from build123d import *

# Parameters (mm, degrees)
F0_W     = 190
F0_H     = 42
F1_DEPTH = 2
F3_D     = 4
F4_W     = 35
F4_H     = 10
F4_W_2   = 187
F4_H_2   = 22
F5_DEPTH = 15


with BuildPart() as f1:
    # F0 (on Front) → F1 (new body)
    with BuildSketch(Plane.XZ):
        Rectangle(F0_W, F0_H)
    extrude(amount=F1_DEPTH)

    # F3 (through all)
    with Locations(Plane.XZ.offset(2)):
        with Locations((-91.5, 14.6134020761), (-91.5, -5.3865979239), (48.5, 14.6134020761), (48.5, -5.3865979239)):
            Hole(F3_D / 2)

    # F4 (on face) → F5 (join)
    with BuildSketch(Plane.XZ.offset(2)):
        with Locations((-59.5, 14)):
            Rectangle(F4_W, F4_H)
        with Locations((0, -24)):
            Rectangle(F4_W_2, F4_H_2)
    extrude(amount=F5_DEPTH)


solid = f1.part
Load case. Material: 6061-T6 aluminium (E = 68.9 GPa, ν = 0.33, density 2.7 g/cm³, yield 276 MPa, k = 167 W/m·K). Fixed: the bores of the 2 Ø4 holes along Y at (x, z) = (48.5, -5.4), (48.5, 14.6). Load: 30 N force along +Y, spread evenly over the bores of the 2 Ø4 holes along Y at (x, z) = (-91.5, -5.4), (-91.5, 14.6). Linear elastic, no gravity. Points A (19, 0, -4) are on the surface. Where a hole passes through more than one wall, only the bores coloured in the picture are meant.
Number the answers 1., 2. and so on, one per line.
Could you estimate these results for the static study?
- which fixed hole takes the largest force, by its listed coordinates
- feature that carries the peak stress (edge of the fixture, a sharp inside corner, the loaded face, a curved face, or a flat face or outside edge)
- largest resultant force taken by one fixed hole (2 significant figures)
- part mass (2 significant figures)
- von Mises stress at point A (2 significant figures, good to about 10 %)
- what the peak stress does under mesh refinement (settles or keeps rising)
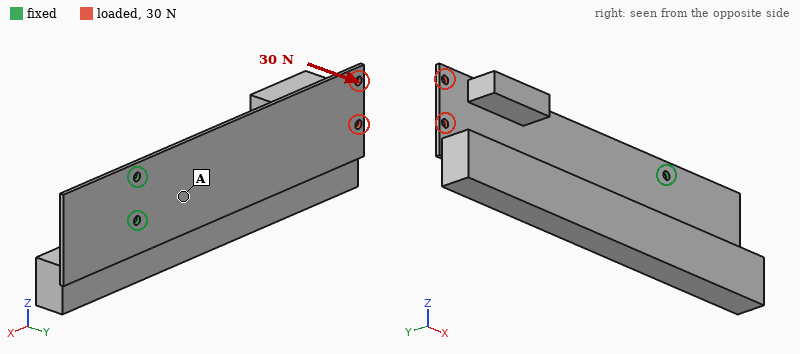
1. (48.5, -5.4)
2. edge of the fixture
3. 19 N
4. 220 g
5. 12 MPa
6. keeps rising
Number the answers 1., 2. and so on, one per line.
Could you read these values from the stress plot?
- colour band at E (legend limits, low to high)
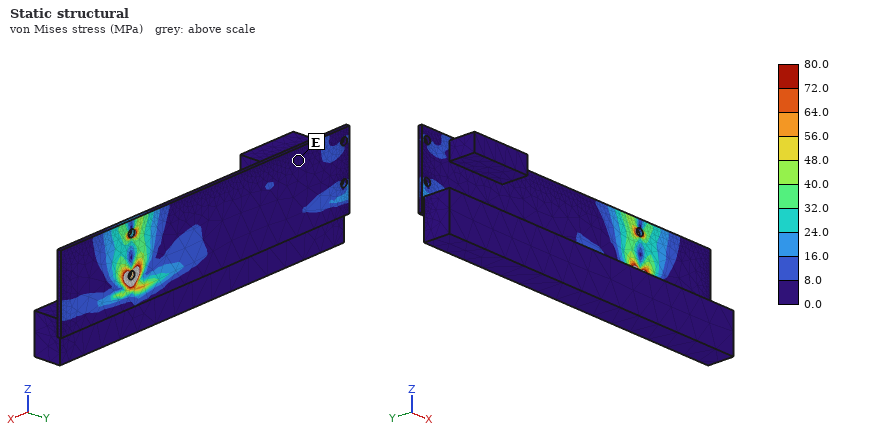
1. 0.0 to 8.0 MPa
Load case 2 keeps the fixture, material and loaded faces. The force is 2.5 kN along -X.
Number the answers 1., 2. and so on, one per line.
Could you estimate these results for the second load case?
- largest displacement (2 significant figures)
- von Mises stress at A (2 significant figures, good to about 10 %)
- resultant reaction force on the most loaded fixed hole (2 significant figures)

1. 0.15 mm
2. 23 MPa
3. 1.3 kN
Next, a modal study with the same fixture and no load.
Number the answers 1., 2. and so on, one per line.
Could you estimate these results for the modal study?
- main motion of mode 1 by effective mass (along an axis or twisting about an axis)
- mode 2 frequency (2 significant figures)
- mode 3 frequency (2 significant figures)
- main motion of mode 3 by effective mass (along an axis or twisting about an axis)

1. along Y
2. 330 Hz
3. 770 Hz
4. along Z
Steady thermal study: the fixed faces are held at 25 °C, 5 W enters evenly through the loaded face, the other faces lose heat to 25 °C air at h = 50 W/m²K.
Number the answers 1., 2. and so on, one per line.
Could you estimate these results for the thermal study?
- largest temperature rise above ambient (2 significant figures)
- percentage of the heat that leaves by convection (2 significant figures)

1. 14 K
2. 77 %
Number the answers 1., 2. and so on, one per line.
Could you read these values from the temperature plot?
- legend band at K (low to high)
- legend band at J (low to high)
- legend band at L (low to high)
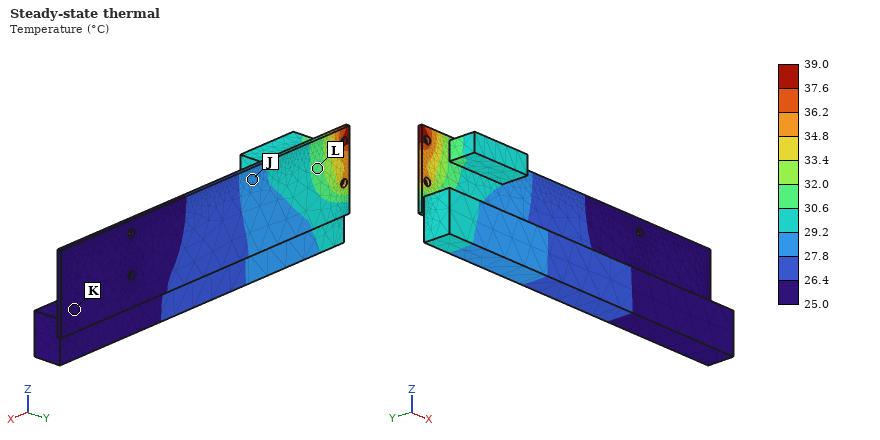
1. 25.0 to 26.4 °C
2. 27.8 to 29.2 °C
3. 30.6 to 32.0 °C
